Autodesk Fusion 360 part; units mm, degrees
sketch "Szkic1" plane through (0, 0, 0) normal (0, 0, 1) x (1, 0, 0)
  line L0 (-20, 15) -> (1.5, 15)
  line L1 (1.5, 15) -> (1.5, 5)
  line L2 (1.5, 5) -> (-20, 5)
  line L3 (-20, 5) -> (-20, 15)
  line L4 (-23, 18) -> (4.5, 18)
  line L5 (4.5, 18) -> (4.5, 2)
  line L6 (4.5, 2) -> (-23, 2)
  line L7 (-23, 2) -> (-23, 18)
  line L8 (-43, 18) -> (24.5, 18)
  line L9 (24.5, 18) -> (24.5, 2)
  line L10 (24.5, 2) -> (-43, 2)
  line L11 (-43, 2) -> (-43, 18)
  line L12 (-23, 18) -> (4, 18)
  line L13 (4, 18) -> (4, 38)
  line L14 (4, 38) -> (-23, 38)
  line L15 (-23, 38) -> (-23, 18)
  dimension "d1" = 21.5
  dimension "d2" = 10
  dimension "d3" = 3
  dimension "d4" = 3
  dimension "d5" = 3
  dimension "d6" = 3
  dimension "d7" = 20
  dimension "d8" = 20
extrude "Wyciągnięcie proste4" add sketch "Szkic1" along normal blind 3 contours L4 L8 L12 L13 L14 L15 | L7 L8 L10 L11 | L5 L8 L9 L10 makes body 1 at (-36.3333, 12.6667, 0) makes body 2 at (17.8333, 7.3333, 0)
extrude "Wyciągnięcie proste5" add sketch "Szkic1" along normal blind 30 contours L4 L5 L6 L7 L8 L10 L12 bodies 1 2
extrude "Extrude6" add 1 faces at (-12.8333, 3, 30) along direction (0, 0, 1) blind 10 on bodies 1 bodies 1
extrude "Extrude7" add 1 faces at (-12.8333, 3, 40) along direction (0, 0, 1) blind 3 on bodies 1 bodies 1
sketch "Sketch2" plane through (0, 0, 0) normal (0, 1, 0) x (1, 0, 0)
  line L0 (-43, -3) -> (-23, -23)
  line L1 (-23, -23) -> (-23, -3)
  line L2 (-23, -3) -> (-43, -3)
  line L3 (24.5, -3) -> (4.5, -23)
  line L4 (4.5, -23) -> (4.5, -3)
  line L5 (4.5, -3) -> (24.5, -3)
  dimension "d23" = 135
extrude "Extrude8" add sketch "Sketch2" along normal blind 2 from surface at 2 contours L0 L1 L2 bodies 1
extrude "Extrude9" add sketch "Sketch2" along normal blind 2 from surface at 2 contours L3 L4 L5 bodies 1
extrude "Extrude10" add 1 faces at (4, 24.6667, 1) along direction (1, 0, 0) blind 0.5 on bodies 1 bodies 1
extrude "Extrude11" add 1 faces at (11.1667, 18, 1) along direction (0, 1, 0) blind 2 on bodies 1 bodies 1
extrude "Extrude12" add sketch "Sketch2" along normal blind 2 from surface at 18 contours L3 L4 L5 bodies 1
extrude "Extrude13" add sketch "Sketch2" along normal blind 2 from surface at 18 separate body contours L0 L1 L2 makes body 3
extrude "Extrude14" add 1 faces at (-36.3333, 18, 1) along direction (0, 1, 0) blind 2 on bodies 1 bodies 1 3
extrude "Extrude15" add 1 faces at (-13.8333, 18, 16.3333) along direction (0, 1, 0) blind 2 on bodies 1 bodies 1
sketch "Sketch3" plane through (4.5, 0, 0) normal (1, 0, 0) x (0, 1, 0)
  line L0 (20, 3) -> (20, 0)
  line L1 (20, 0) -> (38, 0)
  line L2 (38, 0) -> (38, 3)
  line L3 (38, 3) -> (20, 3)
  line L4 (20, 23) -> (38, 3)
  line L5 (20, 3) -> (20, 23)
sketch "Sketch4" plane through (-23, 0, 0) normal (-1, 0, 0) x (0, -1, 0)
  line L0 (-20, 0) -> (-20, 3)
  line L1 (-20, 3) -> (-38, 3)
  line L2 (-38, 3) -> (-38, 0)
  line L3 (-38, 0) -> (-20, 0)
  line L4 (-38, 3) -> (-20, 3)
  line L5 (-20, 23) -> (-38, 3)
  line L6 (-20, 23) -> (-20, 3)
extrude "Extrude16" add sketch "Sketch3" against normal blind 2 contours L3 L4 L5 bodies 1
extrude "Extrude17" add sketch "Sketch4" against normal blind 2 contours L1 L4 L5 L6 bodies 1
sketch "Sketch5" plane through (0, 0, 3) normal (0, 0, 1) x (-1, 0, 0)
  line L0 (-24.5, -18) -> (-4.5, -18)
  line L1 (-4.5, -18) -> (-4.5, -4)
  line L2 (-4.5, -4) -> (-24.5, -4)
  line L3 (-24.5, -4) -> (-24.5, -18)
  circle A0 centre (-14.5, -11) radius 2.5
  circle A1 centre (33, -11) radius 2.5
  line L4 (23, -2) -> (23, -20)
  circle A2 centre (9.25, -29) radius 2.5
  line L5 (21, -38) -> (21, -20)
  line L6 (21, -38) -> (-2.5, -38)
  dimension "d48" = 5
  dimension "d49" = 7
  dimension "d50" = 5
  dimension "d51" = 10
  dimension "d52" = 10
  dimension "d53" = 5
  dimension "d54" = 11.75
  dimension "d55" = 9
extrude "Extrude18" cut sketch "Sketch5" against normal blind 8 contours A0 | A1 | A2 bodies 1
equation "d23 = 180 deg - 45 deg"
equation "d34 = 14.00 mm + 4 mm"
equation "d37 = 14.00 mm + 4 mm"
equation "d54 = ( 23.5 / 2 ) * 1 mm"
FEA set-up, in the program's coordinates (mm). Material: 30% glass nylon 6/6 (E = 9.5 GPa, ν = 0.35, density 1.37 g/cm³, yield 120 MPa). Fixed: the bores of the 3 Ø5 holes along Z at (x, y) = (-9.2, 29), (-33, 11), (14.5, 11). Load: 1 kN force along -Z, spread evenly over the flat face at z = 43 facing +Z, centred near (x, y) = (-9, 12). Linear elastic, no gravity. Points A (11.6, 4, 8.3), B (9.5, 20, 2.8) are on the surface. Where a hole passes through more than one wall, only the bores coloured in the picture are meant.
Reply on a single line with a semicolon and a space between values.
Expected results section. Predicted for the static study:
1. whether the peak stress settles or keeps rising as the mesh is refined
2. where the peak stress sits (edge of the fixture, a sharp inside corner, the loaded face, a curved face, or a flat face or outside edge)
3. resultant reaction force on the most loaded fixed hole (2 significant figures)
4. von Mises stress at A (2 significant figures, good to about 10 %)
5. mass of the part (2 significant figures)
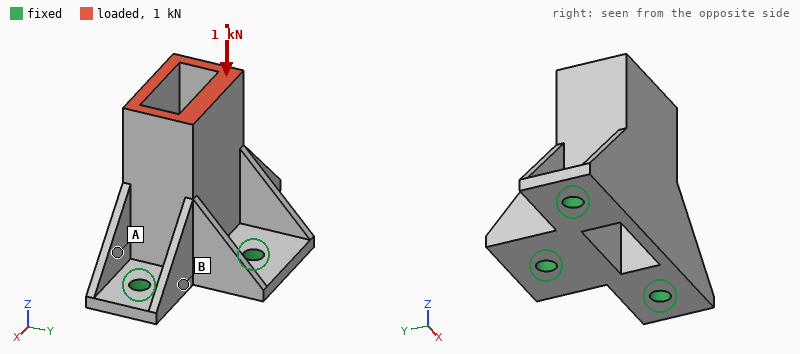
keeps rising; edge of the fixture; 490 N; 14 MPa; 24 g
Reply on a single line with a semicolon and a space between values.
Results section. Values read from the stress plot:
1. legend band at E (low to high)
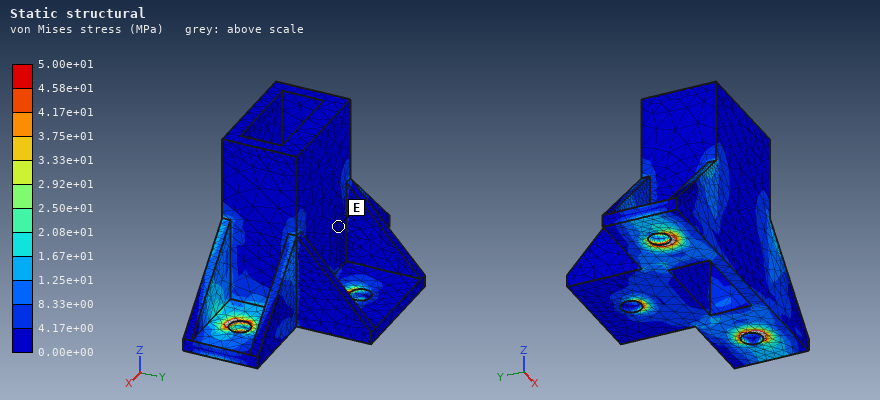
0.00e+00 to 4.17e+00 MPa
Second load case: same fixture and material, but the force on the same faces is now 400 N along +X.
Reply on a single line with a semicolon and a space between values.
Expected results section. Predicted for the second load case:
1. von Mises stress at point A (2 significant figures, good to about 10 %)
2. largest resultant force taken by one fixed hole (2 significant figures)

11 MPa; 400 N
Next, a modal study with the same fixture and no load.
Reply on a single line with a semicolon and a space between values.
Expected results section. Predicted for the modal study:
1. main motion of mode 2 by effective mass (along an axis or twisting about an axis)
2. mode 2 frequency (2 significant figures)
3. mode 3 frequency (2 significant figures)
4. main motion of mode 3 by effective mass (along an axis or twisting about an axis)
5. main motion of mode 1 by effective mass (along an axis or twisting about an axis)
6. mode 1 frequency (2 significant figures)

along X; 3900 Hz; 5000 Hz; along Z; along Y; 1800 Hz
